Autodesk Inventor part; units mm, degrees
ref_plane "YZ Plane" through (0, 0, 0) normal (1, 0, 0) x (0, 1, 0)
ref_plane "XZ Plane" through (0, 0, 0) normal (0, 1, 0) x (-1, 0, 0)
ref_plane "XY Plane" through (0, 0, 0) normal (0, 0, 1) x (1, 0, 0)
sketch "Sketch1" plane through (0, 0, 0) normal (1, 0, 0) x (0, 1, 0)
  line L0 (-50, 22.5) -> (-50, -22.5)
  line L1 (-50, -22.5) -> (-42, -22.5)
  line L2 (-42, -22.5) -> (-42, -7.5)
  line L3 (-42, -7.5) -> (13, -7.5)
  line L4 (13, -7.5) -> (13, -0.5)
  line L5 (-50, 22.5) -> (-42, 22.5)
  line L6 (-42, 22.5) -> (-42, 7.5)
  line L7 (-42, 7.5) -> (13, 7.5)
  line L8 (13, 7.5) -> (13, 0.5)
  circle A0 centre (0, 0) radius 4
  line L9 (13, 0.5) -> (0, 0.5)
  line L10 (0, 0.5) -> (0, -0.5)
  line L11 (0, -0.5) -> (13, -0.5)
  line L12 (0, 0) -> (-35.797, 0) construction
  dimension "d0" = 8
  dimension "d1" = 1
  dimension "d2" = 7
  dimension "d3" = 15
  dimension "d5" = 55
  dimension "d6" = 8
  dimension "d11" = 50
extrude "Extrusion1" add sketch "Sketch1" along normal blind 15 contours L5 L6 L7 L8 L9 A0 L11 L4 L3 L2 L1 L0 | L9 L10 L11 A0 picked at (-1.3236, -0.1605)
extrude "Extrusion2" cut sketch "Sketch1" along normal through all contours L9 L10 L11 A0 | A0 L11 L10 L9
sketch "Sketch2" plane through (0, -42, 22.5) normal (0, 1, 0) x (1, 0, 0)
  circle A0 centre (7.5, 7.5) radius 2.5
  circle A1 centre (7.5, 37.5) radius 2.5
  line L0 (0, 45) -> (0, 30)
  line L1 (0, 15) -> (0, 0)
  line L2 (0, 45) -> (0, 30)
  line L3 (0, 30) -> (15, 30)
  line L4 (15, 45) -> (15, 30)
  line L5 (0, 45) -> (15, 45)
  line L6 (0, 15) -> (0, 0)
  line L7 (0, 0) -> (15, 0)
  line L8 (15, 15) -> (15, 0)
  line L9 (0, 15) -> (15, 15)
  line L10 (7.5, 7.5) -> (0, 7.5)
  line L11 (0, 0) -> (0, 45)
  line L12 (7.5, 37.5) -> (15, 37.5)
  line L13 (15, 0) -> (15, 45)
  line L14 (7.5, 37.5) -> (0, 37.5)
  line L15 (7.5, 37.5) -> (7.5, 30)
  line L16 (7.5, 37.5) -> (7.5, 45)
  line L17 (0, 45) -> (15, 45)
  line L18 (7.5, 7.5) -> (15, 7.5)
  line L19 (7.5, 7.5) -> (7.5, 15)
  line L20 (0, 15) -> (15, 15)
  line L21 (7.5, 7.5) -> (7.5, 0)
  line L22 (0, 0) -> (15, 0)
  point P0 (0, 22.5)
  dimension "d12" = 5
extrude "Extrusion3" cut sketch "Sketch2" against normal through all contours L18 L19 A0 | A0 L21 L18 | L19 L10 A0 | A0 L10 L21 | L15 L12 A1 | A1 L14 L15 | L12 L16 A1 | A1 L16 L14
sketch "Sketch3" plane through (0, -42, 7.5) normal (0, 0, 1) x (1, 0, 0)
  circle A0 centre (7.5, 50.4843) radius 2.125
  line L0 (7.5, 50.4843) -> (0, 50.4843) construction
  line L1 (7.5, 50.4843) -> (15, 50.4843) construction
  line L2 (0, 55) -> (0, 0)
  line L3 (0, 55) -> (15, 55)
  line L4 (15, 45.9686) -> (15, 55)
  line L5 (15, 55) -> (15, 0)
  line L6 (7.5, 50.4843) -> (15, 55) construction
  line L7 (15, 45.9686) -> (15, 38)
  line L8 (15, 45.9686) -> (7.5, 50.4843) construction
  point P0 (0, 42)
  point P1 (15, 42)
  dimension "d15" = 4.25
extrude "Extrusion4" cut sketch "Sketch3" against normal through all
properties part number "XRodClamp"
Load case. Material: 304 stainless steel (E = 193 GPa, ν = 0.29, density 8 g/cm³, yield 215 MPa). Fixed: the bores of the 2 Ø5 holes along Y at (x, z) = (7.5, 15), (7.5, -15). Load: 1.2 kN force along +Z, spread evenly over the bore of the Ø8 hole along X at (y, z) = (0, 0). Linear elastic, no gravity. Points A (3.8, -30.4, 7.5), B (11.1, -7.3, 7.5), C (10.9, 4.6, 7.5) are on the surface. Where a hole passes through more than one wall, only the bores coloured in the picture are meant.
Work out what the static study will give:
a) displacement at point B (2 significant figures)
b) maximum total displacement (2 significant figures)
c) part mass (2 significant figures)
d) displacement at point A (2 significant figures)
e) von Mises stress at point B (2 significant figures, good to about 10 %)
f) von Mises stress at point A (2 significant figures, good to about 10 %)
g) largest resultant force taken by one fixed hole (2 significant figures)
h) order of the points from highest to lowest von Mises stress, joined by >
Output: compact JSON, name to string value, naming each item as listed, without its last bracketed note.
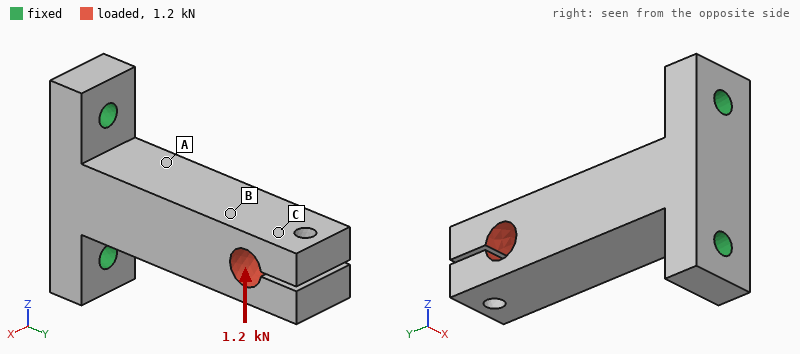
{"displacement at point B": "49 µm", "maximum total displacement": "94 µm", "part mass": "130 g", "displacement at point A": "14 µm", "von Mises stress at point B": "24 MPa", "von Mises stress at point A": "64 MPa", "largest resultant force taken by one fixed hole": "2.5 kN", "order of the points from highest to lowest von Mises stress, joined by >": "A > B > C"}
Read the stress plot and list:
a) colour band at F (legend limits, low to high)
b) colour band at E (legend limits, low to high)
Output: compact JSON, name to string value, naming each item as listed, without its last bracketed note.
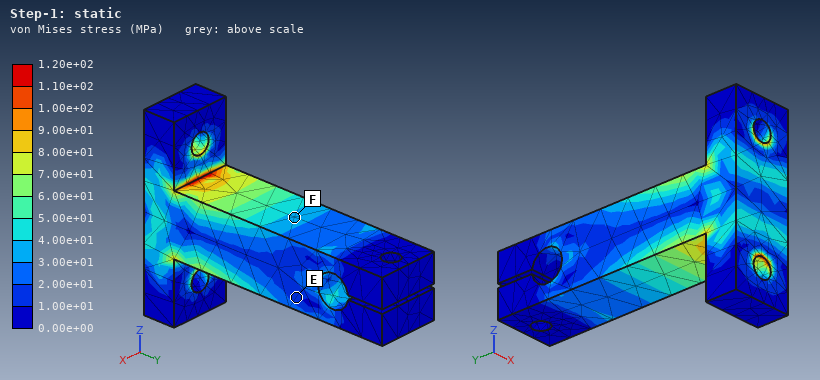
{"colour band at F": "3.00e+01 to 4.00e+01 MPa", "colour band at E": "1.00e+01 to 2.00e+01 MPa"}
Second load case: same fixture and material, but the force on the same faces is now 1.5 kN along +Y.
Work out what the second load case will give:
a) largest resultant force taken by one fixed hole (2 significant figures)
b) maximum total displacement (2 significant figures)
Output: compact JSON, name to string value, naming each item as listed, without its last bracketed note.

{"largest resultant force taken by one fixed hole": "780 N", "maximum total displacement": "11 µm"}
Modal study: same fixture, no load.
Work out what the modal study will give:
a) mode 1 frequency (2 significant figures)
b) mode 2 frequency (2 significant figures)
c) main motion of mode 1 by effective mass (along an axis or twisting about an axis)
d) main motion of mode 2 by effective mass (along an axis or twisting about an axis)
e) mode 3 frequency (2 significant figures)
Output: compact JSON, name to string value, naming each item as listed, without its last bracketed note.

{"mode 1 frequency": "2300 Hz", "mode 2 frequency": "3200 Hz", "main motion of mode 1 by effective mass": "along X", "main motion of mode 2 by effective mass": "along Z", "mode 3 frequency": "7300 Hz"}
